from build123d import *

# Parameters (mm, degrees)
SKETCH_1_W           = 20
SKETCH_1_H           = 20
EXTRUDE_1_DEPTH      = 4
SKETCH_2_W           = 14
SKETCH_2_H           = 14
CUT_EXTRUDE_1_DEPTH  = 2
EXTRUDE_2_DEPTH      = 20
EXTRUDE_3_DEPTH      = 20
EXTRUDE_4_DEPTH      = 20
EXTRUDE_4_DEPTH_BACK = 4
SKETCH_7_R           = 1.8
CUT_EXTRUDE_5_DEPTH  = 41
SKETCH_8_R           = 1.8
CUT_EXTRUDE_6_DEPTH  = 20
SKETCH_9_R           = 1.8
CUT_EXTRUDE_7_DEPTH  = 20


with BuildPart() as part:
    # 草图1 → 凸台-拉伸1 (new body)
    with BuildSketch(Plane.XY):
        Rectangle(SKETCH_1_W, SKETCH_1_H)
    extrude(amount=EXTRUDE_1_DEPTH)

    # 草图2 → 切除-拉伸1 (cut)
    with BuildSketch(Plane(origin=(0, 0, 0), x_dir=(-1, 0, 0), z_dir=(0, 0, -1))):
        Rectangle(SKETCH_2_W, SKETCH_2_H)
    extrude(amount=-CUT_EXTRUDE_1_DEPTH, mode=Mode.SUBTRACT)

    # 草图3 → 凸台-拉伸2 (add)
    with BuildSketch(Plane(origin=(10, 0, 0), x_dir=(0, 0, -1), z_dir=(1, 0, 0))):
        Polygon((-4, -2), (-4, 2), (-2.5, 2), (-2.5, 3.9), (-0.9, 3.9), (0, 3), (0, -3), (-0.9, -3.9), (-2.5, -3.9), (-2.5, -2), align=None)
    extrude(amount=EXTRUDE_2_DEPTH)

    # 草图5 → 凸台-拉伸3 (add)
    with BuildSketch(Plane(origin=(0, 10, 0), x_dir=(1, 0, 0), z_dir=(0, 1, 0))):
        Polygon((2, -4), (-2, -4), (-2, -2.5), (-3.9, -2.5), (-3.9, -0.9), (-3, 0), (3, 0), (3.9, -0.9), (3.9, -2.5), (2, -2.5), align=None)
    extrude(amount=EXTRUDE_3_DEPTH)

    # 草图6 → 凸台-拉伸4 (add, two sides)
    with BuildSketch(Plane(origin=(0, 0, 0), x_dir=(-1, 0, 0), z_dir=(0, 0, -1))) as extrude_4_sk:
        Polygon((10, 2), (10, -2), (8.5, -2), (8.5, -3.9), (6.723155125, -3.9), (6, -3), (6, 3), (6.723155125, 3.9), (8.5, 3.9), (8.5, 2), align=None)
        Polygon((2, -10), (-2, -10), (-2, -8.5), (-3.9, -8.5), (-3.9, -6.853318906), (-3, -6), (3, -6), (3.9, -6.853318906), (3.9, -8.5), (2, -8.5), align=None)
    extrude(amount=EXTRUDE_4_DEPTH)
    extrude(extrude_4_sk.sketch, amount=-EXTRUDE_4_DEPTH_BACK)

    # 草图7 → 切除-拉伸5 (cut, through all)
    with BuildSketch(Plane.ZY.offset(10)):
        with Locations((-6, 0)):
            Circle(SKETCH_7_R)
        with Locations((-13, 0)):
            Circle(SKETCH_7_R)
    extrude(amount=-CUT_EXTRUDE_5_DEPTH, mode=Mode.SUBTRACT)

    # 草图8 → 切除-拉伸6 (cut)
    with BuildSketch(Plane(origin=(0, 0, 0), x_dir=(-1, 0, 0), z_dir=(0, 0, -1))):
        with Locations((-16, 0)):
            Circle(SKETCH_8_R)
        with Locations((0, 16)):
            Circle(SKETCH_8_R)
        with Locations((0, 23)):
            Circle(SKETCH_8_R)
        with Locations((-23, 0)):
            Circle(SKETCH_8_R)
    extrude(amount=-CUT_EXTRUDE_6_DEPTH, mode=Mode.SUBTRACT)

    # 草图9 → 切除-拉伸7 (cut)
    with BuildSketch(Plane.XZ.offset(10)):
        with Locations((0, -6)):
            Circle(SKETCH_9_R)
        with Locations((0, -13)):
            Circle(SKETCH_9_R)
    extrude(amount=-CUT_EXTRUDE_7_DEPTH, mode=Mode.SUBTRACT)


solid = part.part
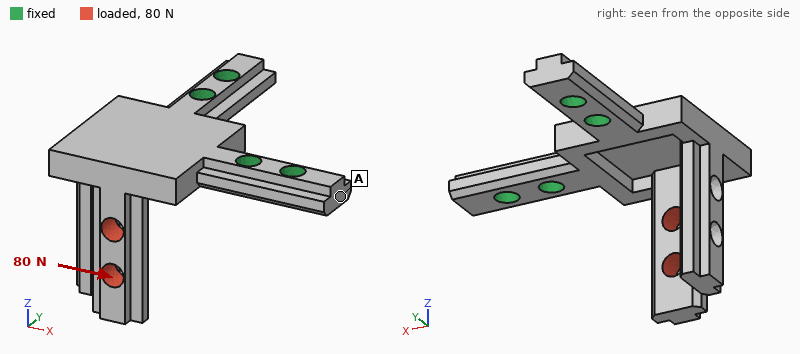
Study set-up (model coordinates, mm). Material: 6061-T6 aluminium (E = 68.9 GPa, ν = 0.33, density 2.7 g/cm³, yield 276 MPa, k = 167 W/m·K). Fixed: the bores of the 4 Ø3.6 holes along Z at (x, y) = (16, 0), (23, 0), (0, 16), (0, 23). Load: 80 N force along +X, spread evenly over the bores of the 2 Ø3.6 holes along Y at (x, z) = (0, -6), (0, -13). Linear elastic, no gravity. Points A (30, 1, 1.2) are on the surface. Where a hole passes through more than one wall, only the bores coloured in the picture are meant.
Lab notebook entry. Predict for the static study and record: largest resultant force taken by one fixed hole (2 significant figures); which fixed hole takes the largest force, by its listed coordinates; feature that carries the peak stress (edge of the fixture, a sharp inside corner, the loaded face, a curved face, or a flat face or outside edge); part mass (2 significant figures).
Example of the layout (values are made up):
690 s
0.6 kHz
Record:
90 N
(16, 0)
a flat face or outside edge
7.8 g
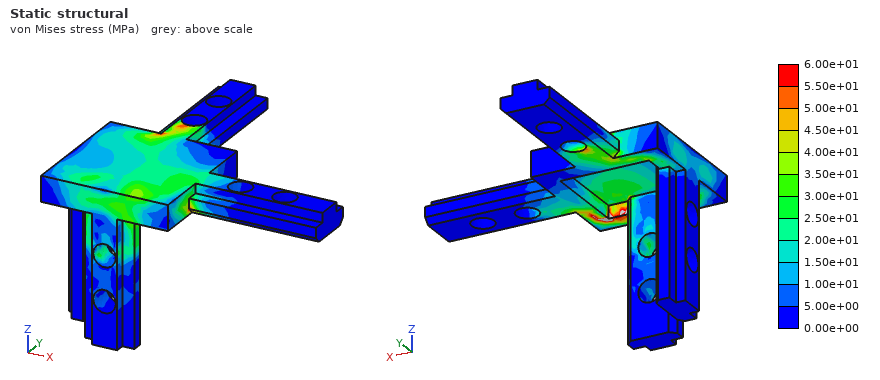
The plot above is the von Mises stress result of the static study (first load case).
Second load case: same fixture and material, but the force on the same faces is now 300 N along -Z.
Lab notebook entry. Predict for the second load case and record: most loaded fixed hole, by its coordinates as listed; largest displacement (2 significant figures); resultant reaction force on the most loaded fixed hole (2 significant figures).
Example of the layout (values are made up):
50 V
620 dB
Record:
(16, 0)
0.40 mm
260 N
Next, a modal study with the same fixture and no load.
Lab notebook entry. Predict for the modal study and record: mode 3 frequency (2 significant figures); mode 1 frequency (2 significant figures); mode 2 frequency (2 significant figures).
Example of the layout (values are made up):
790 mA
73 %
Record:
4400 Hz
2400 Hz
3500 Hz
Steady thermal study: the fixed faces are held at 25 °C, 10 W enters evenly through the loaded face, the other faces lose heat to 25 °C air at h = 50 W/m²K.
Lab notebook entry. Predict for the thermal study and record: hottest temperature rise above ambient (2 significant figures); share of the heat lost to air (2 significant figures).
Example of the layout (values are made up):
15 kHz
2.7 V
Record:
54 K
19 %
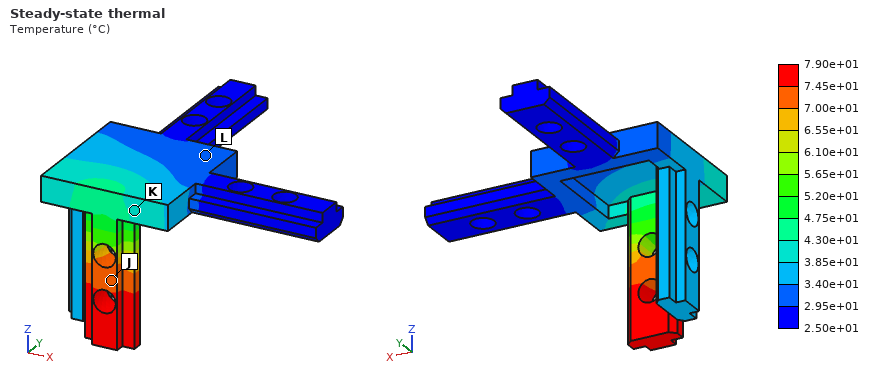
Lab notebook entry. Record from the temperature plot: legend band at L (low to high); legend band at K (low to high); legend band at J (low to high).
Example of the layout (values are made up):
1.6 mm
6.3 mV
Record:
2.95e+01 to 3.40e+01 °C
3.85e+01 to 4.30e+01 °C
7.00e+01 to 7.45e+01 °C
